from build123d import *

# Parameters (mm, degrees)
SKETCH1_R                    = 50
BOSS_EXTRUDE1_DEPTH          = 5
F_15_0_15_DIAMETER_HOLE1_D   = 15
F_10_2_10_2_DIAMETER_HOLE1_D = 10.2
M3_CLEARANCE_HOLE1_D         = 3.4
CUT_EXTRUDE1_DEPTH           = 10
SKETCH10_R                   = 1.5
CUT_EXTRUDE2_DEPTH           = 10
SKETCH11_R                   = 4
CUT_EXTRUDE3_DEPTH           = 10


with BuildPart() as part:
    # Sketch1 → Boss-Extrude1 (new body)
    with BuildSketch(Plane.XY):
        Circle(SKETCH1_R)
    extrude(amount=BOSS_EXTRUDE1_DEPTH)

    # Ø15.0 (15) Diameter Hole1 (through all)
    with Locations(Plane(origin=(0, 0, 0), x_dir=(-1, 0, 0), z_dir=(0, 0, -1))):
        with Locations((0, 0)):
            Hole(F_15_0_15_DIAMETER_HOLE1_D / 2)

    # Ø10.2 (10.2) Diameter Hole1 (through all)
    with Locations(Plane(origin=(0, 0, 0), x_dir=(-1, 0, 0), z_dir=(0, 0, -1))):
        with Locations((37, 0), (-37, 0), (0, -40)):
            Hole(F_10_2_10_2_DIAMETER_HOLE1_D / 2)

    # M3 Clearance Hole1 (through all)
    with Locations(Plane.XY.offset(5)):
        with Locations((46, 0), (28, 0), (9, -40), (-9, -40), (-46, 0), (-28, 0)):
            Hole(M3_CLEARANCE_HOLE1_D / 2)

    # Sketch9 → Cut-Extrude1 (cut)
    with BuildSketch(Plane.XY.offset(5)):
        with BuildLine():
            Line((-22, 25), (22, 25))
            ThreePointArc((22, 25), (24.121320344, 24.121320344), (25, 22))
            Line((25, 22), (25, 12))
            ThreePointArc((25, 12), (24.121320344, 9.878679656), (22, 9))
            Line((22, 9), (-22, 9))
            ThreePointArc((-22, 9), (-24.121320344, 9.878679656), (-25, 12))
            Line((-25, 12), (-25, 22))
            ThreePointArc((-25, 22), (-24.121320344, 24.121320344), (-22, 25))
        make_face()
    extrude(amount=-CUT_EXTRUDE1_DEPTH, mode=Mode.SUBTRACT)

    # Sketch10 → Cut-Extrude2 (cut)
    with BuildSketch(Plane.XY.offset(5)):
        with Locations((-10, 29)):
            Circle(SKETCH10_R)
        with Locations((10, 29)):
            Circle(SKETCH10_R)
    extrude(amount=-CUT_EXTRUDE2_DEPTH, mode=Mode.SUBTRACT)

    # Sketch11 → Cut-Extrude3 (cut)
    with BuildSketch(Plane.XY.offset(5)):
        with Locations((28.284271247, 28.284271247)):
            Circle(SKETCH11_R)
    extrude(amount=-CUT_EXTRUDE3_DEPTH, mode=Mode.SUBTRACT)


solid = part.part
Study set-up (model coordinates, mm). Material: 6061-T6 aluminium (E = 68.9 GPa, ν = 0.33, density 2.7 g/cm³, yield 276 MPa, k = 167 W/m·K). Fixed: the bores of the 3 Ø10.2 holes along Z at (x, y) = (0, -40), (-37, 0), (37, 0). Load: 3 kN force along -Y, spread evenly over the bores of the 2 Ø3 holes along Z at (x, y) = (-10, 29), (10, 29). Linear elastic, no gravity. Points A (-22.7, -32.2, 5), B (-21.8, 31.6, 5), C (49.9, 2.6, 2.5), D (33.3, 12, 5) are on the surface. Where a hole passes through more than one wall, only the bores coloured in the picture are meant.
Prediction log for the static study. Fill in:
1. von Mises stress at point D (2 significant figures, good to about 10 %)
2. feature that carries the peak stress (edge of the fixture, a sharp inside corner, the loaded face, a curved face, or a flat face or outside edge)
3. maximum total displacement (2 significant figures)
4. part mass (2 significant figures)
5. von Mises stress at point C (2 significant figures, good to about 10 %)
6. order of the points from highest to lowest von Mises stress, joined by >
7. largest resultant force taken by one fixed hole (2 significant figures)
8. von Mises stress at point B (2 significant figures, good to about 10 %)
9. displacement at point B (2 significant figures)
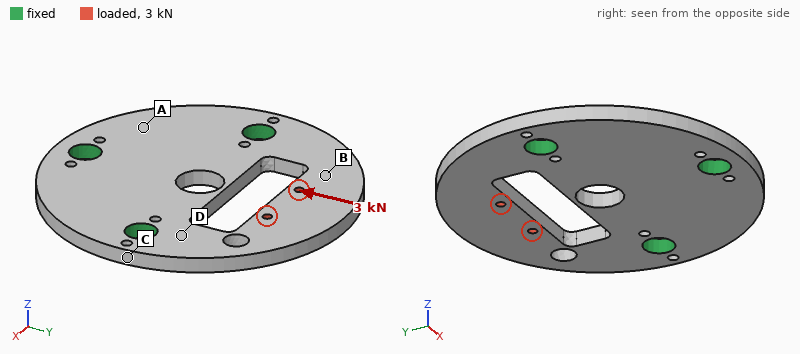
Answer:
25 MPa
a curved face
39 µm
88 g
15 MPa
B > D > C > A
1.7 kN
36 MPa
17 µm
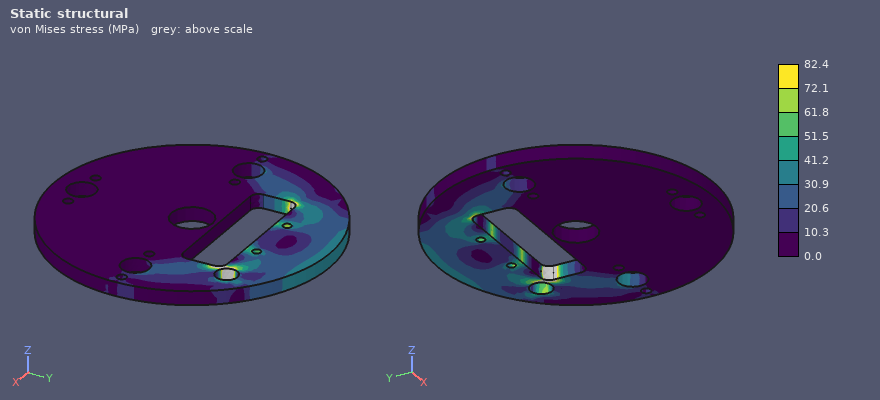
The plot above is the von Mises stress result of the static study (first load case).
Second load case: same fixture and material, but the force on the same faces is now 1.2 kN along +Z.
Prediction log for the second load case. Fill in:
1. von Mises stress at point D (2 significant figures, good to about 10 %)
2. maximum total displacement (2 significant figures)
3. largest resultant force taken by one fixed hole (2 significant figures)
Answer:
120 MPa
0.67 mm
650 N
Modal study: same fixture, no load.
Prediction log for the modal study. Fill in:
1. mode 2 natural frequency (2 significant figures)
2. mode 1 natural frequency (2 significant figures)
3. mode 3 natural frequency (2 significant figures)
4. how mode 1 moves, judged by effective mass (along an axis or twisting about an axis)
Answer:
4300 Hz
1600 Hz
6600 Hz
along Z
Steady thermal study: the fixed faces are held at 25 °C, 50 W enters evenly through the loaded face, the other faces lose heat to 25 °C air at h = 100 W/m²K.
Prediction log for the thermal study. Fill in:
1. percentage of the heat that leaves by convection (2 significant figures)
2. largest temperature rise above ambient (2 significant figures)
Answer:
39 %
65 K
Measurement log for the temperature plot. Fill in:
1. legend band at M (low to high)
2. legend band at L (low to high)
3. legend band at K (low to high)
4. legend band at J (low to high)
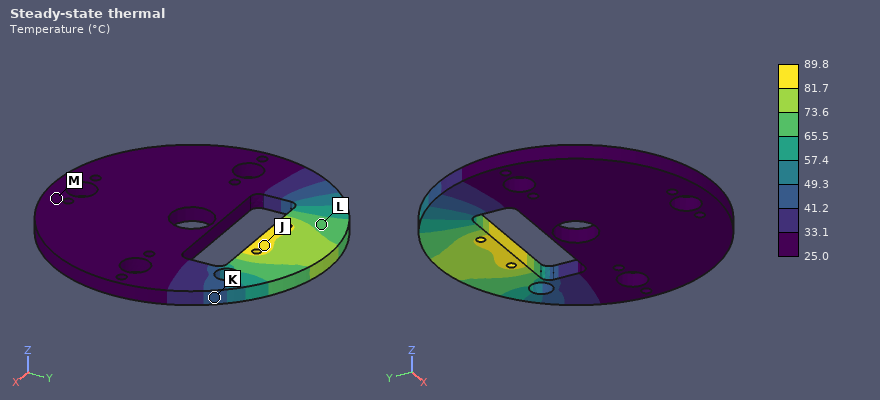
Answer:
25.0 to 33.1 °C
65.5 to 73.6 °C
41.2 to 49.3 °C
81.7 to 89.8 °C
